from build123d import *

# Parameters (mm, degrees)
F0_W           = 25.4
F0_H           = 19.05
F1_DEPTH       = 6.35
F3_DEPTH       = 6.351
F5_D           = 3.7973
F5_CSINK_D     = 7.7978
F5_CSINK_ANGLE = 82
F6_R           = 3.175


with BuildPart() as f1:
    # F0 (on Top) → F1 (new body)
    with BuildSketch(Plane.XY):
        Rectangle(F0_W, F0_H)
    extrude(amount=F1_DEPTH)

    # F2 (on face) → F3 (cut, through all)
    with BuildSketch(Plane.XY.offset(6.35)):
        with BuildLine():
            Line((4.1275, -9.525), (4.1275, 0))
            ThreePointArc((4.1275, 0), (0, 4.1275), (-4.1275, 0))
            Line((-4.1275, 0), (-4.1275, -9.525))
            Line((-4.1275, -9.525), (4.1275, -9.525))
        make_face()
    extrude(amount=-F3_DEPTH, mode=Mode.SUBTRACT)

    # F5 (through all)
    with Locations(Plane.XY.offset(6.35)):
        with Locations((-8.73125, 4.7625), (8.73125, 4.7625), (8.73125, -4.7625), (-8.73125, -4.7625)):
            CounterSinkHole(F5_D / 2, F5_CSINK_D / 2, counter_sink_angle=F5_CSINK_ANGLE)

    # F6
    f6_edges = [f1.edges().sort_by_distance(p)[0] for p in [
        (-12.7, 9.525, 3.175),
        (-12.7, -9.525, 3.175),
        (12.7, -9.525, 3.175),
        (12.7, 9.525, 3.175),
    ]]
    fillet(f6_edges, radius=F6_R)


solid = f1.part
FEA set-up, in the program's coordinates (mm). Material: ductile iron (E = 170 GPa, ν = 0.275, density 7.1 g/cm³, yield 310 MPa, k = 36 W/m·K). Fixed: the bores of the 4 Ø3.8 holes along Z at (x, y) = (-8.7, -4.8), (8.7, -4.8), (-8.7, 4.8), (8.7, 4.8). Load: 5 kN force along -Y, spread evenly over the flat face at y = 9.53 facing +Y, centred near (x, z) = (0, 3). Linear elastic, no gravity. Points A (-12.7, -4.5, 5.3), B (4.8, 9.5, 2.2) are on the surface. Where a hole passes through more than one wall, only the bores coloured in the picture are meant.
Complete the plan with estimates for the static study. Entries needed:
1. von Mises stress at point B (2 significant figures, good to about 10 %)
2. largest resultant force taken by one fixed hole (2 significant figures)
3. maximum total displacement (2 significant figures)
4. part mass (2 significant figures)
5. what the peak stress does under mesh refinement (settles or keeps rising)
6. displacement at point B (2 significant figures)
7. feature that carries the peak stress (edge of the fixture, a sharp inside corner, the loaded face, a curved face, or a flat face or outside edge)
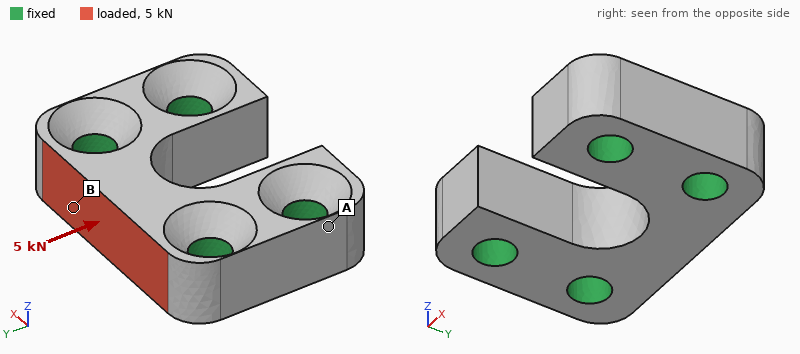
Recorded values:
46 MPa
2.0 kN
5.5 µm
14 g
keeps rising
3.1 µm
edge of the fixture
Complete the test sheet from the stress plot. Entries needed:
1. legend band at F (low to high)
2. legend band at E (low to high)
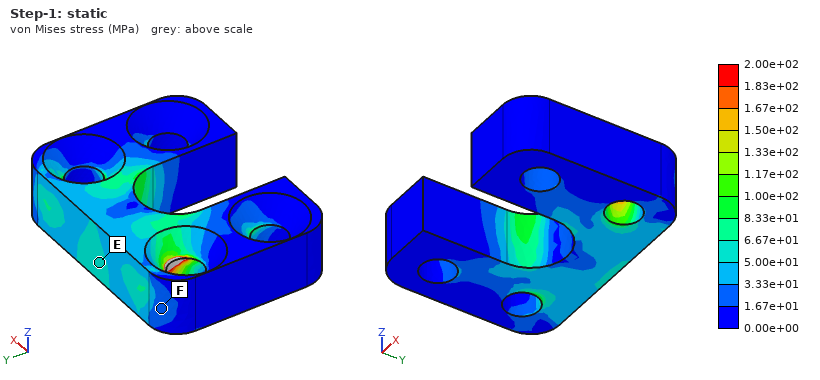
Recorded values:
1.67e+01 to 3.33e+01 MPa
5.00e+01 to 6.67e+01 MPa
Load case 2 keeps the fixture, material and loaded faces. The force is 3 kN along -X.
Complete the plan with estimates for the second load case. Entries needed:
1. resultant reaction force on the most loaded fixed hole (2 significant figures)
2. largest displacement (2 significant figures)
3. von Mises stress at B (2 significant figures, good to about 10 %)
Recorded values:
1.6 kN
2.2 µm
45 MPa
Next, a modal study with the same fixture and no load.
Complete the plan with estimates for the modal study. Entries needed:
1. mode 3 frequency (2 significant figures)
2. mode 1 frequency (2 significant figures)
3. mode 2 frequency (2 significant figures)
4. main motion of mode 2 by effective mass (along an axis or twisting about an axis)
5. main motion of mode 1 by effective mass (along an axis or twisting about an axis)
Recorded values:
98 kHz
64 kHz
89 kHz
along Y
along Z
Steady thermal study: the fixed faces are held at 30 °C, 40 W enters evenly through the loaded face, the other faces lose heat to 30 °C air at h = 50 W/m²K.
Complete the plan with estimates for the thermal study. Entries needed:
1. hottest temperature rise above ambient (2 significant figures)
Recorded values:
70 K
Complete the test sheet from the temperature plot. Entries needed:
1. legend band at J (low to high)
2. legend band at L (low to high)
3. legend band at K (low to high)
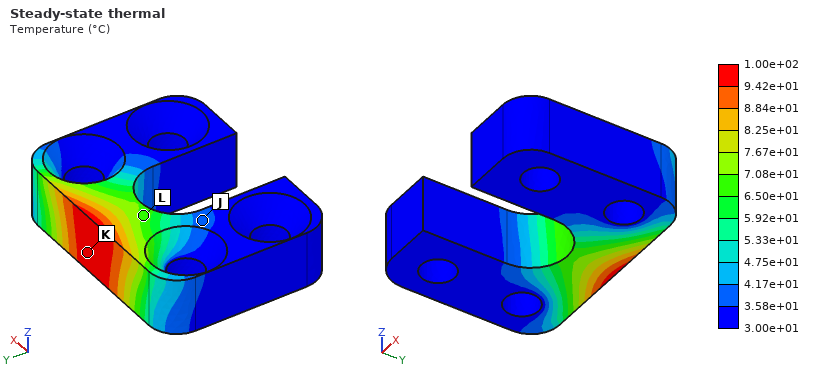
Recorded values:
3.58e+01 to 4.17e+01 °C
6.50e+01 to 7.08e+01 °C
9.42e+01 to 1.00e+02 °C
